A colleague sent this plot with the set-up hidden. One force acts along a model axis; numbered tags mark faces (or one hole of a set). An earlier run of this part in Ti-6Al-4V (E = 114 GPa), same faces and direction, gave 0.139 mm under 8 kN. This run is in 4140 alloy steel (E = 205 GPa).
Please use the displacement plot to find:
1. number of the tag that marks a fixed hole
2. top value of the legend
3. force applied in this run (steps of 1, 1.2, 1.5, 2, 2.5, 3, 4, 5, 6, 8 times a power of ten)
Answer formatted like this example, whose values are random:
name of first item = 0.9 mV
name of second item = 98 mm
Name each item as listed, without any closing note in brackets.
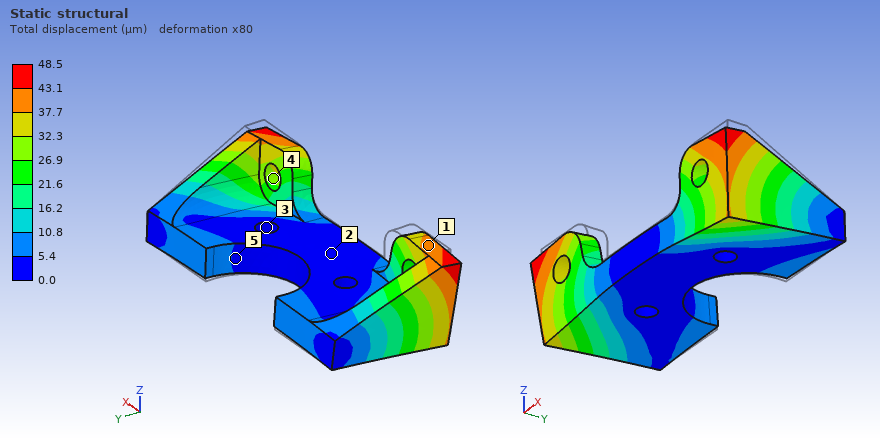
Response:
number of the tag that marks a fixed hole = 3
top value of the legend = 48.5 µm
force applied in this run = 5 kN
